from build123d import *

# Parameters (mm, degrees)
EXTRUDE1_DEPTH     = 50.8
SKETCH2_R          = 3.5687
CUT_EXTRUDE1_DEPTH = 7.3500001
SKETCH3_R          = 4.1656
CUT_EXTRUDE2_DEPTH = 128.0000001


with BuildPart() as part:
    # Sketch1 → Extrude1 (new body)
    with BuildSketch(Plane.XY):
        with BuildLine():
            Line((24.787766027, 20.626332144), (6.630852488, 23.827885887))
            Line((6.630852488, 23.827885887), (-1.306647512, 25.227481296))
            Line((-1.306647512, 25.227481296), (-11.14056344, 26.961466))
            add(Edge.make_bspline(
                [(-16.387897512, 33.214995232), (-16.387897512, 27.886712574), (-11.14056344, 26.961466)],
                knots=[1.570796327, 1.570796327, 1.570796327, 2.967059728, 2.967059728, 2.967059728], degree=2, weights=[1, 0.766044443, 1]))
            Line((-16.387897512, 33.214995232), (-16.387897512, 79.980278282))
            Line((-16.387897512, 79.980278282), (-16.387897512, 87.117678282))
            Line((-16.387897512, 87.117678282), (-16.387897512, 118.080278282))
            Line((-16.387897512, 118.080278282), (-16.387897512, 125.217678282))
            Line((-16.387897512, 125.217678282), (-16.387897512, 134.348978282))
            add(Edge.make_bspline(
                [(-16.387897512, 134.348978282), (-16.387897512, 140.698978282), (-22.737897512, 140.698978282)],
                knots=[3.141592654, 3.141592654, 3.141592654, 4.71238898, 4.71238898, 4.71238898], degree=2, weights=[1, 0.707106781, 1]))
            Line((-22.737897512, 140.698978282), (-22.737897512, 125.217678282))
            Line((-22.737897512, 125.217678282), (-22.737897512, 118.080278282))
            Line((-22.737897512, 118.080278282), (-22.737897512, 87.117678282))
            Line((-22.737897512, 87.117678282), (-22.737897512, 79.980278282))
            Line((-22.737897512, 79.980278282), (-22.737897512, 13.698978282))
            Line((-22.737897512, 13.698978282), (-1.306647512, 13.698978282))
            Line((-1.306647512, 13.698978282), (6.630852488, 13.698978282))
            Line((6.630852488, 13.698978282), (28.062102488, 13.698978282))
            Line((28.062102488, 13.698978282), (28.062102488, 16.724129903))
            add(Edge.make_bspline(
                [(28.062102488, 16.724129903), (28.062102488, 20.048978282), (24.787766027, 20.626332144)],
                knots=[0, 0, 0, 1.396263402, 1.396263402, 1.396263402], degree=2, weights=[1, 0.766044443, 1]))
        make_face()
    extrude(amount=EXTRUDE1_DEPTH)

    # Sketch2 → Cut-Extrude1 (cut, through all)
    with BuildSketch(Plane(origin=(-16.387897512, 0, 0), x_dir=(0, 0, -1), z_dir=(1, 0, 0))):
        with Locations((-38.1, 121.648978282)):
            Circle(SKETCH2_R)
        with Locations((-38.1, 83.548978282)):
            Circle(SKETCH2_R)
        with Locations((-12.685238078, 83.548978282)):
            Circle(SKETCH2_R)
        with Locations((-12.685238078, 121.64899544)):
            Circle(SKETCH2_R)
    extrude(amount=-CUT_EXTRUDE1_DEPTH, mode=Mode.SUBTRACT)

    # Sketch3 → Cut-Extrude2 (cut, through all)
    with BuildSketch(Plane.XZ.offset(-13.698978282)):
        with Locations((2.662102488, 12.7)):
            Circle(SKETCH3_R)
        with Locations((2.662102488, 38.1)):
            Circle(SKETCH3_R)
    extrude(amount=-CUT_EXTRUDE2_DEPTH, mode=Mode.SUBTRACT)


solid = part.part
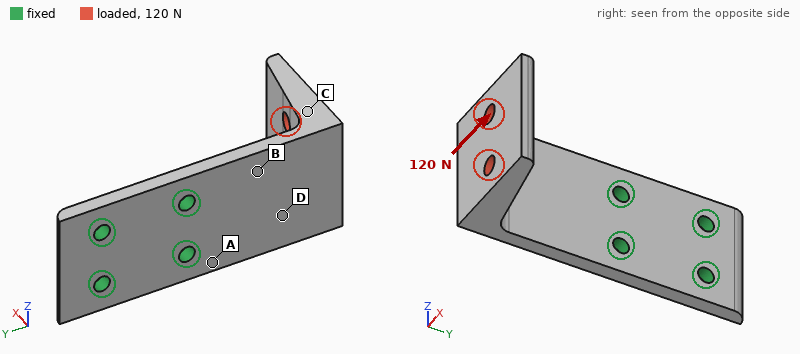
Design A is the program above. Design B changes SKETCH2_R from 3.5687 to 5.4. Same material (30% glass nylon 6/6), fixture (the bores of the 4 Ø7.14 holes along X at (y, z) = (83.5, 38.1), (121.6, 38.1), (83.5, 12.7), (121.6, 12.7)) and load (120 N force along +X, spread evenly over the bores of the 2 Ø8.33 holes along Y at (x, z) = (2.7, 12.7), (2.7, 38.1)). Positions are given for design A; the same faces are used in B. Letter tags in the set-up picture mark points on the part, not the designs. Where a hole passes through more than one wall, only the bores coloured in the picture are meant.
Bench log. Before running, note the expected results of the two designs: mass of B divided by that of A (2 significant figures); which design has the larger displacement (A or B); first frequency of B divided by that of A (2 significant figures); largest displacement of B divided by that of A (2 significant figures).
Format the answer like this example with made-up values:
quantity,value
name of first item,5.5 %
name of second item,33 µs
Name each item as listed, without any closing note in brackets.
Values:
quantity,value
mass of B divided by that of A,0.98
which design has the larger displacement,A
first frequency of B divided by that of A,1.1
largest displacement of B divided by that of A,0.91
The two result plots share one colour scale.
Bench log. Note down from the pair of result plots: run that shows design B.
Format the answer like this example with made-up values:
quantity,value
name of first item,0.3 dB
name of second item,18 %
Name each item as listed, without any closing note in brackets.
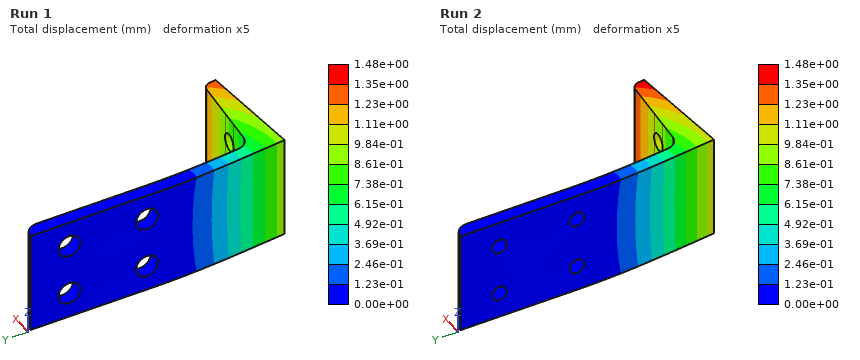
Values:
quantity,value
run that shows design B,Run 1
